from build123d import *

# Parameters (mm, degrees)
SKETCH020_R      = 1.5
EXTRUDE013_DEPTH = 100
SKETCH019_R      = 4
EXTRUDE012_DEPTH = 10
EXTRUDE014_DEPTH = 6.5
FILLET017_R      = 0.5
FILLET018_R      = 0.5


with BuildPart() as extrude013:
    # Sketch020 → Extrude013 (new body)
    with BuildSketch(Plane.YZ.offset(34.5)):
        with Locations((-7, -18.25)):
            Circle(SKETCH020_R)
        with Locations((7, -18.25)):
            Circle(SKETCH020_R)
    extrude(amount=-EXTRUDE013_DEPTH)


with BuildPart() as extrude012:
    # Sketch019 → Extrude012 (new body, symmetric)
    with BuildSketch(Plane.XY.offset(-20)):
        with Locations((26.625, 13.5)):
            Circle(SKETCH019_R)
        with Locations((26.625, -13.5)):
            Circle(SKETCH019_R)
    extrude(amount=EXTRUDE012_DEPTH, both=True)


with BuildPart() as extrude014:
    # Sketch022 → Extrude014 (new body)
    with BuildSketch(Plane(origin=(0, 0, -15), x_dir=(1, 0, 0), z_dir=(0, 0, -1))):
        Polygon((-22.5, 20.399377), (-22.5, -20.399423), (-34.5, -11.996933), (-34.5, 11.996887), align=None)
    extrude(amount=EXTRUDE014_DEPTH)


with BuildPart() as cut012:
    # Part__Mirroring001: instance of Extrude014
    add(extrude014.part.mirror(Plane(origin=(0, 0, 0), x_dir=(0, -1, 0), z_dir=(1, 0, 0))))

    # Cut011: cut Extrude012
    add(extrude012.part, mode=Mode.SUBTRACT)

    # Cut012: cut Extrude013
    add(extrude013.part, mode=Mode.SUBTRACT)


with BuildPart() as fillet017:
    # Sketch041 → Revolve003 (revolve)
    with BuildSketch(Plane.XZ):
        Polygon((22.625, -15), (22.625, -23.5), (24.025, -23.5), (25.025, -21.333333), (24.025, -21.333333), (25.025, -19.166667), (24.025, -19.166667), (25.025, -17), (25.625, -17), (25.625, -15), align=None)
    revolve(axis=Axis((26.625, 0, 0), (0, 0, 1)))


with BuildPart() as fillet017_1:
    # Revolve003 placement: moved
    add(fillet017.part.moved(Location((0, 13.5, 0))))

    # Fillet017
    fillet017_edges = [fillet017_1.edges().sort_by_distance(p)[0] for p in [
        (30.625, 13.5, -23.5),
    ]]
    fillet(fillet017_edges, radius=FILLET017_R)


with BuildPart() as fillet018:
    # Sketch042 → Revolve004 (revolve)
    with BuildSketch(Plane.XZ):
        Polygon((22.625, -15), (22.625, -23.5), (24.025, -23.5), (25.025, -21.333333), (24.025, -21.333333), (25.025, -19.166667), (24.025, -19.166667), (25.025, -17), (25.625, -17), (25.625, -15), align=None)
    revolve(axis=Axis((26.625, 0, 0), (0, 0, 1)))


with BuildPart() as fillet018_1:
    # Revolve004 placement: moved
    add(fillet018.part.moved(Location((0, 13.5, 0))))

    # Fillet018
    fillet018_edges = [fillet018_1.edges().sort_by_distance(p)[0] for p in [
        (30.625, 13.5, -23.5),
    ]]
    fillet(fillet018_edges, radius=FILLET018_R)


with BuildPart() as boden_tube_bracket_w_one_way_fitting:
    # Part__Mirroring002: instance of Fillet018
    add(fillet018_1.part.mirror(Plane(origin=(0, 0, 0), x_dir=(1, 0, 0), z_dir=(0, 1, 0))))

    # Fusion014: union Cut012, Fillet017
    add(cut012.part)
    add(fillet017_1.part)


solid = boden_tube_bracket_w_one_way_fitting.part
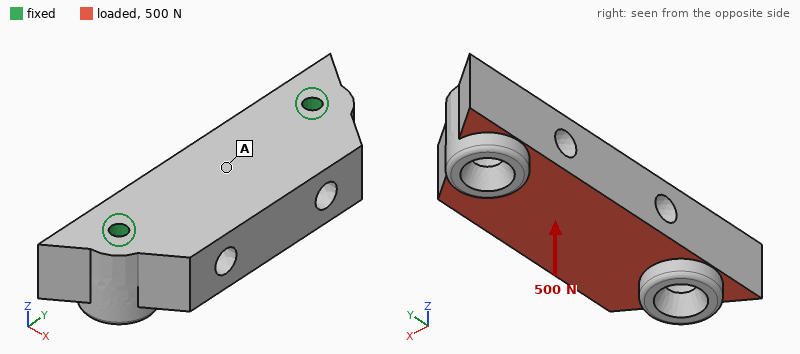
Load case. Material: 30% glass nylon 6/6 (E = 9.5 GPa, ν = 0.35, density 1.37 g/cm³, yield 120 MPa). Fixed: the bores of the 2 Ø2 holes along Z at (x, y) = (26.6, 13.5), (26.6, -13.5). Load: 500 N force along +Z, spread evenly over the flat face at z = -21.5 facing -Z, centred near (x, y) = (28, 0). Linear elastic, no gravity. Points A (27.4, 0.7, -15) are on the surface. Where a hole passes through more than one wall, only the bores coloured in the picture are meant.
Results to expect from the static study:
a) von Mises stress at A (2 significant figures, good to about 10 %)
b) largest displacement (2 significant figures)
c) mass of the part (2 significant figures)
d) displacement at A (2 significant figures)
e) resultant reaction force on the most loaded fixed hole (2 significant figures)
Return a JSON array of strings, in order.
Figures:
["11 MPa", "0.11 mm", "3.3 g", "0.052 mm", "300 N"]
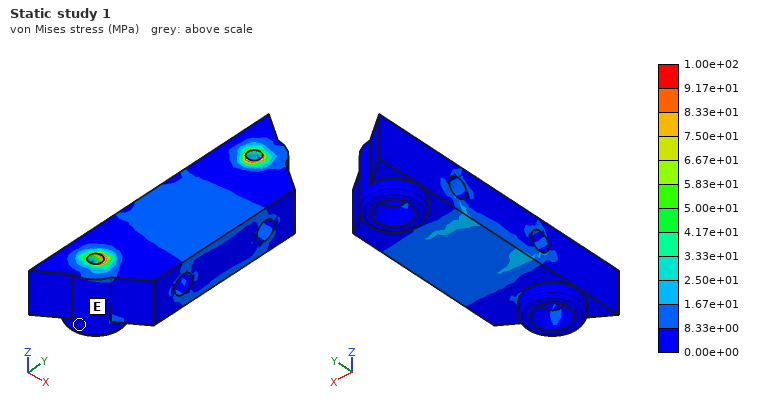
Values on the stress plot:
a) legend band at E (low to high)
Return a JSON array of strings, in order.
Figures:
["0.00e+00 to 8.33e+00 MPa"]
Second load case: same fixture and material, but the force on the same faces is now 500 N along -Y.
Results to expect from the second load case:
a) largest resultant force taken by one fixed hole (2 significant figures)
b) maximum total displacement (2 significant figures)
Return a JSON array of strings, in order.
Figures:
["270 N", "20 µm"]
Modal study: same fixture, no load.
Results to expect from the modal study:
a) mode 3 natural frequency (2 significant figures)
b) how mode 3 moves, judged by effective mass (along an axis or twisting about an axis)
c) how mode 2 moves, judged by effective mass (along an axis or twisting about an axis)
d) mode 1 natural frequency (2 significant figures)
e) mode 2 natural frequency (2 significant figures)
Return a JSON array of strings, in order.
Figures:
["16 kHz", "along X", "along Z", "6400 Hz", "12 kHz"]
